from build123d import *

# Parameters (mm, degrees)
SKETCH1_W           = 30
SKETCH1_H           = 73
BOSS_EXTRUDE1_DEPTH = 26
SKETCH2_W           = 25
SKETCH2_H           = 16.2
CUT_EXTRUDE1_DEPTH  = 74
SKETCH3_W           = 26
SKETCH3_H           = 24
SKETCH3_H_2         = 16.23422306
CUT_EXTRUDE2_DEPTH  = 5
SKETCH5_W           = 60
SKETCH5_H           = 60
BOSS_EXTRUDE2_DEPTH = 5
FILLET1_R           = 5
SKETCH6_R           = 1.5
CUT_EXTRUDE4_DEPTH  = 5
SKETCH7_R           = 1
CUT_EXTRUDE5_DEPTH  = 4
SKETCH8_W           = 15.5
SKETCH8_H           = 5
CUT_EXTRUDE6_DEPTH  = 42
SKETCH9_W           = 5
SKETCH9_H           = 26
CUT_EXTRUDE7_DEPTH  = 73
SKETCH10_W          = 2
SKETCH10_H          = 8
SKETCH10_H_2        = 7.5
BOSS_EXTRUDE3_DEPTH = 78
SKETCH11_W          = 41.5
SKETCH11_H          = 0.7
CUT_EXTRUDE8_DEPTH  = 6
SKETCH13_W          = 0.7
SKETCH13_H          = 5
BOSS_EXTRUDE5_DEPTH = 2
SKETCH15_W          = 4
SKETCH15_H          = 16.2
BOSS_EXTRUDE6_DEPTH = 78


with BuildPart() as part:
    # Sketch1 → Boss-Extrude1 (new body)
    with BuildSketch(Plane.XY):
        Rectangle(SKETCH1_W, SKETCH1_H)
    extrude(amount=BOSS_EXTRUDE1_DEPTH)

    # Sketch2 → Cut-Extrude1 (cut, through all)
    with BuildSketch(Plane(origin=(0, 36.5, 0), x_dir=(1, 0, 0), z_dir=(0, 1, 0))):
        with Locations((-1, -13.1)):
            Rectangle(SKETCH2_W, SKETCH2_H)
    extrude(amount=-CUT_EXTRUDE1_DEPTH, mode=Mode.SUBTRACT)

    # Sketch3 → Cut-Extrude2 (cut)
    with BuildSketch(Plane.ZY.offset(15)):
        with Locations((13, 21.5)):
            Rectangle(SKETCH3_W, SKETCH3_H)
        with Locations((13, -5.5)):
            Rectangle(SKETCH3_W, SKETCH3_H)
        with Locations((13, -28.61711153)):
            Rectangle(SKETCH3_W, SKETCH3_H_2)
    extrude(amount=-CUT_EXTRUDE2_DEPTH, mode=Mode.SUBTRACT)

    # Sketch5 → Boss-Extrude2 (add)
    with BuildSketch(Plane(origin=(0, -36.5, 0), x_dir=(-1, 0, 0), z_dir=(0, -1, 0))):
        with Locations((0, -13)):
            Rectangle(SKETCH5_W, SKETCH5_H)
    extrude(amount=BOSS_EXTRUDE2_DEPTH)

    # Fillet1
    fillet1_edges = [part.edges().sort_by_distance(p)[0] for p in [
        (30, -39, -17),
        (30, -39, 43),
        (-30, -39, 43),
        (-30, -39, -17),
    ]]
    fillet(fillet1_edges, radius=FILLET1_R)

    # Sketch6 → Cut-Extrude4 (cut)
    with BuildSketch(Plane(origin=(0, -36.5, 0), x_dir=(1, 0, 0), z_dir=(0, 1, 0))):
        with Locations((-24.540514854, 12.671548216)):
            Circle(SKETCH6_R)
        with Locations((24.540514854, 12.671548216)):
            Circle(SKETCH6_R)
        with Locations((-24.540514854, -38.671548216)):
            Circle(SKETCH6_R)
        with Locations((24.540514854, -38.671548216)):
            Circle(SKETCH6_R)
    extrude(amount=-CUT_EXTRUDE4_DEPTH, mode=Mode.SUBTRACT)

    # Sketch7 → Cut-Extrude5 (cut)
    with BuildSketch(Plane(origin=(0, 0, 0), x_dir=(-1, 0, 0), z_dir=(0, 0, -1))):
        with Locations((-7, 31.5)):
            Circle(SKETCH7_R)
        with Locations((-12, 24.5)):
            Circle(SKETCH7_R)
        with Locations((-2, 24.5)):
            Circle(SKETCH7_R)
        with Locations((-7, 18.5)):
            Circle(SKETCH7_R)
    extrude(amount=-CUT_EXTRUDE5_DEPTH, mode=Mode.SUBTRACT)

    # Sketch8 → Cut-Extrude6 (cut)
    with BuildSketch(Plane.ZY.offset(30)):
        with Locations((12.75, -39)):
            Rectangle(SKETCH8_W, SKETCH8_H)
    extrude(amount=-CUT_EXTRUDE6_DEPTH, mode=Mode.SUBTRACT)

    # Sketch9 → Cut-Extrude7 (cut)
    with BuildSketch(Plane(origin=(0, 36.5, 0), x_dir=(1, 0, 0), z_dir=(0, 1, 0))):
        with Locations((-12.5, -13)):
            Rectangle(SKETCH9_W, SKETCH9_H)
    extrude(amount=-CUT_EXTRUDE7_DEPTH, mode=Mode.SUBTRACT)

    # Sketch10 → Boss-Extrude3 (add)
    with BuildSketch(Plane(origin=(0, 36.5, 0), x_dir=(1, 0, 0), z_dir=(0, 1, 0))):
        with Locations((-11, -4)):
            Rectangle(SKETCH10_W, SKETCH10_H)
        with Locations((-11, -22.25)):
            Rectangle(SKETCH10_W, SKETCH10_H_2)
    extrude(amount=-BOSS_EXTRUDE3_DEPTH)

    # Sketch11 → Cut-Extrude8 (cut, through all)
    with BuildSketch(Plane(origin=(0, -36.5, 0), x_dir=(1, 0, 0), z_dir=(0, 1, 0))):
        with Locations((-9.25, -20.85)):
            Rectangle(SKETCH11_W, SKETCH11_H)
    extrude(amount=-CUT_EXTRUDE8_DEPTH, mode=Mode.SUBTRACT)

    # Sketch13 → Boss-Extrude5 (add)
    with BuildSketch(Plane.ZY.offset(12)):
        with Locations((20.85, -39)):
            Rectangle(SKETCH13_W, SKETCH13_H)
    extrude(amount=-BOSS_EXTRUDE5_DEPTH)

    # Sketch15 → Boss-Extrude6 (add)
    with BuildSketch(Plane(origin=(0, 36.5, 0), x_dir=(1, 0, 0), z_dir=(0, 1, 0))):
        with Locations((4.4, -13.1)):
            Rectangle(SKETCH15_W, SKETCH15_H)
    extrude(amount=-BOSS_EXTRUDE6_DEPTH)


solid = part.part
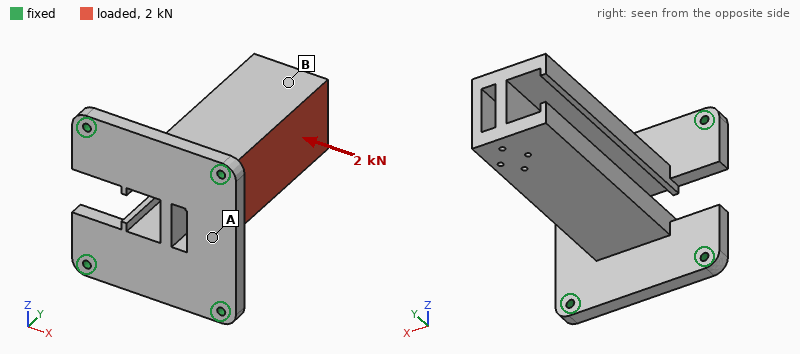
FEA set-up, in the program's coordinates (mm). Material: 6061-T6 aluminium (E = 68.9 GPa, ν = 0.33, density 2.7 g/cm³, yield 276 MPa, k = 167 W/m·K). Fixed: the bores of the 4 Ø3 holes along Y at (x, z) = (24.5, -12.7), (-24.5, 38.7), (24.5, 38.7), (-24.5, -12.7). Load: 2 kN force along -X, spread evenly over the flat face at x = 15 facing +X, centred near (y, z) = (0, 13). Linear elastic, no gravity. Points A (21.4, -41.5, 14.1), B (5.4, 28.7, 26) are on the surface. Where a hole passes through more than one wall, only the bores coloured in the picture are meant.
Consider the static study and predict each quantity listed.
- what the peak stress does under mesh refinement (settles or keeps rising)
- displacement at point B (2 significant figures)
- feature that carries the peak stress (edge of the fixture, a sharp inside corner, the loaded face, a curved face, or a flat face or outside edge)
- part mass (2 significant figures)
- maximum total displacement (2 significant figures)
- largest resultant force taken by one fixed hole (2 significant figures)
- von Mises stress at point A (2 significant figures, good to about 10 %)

keeps rising
0.37 mm
edge of the fixture
120 g
0.43 mm
1.1 kN
43 MPa
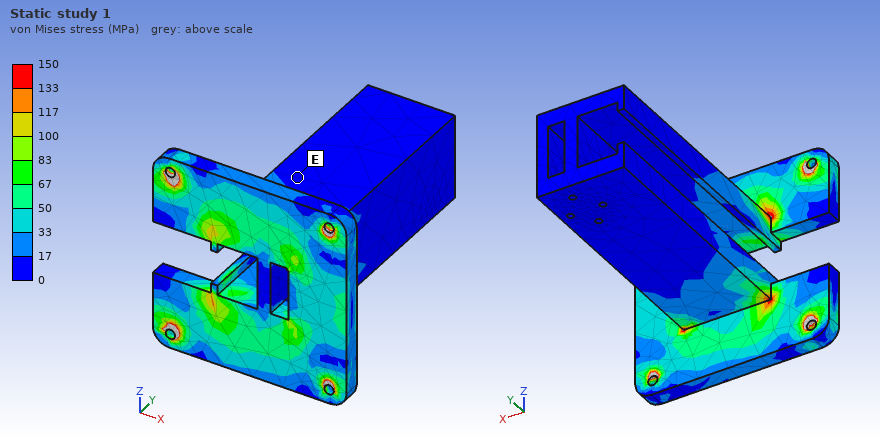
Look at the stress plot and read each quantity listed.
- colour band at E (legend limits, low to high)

0 to 17 MPa
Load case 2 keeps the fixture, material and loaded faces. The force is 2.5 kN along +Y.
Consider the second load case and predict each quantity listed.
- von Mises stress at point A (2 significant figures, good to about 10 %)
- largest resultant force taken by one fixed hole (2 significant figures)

40 MPa
1.1 kN
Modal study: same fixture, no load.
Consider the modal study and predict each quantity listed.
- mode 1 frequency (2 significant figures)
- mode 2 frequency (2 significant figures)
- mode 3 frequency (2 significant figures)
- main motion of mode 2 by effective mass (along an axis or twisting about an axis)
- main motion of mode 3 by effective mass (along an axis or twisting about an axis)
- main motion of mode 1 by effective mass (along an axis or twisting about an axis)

1500 Hz
1600 Hz
3500 Hz
along Z
along Y
along X
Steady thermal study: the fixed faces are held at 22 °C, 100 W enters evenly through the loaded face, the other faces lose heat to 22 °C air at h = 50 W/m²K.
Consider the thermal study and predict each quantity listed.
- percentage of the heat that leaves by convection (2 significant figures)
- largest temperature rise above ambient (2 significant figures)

35 %
68 K
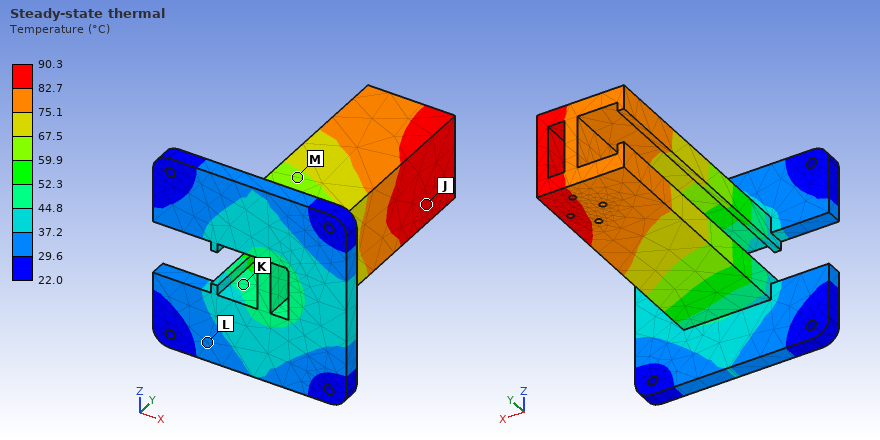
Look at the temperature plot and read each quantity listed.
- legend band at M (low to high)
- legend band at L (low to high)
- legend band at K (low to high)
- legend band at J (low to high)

59.9 to 67.5 °C
29.6 to 37.2 °C
44.8 to 52.3 °C
82.7 to 90.3 °C
